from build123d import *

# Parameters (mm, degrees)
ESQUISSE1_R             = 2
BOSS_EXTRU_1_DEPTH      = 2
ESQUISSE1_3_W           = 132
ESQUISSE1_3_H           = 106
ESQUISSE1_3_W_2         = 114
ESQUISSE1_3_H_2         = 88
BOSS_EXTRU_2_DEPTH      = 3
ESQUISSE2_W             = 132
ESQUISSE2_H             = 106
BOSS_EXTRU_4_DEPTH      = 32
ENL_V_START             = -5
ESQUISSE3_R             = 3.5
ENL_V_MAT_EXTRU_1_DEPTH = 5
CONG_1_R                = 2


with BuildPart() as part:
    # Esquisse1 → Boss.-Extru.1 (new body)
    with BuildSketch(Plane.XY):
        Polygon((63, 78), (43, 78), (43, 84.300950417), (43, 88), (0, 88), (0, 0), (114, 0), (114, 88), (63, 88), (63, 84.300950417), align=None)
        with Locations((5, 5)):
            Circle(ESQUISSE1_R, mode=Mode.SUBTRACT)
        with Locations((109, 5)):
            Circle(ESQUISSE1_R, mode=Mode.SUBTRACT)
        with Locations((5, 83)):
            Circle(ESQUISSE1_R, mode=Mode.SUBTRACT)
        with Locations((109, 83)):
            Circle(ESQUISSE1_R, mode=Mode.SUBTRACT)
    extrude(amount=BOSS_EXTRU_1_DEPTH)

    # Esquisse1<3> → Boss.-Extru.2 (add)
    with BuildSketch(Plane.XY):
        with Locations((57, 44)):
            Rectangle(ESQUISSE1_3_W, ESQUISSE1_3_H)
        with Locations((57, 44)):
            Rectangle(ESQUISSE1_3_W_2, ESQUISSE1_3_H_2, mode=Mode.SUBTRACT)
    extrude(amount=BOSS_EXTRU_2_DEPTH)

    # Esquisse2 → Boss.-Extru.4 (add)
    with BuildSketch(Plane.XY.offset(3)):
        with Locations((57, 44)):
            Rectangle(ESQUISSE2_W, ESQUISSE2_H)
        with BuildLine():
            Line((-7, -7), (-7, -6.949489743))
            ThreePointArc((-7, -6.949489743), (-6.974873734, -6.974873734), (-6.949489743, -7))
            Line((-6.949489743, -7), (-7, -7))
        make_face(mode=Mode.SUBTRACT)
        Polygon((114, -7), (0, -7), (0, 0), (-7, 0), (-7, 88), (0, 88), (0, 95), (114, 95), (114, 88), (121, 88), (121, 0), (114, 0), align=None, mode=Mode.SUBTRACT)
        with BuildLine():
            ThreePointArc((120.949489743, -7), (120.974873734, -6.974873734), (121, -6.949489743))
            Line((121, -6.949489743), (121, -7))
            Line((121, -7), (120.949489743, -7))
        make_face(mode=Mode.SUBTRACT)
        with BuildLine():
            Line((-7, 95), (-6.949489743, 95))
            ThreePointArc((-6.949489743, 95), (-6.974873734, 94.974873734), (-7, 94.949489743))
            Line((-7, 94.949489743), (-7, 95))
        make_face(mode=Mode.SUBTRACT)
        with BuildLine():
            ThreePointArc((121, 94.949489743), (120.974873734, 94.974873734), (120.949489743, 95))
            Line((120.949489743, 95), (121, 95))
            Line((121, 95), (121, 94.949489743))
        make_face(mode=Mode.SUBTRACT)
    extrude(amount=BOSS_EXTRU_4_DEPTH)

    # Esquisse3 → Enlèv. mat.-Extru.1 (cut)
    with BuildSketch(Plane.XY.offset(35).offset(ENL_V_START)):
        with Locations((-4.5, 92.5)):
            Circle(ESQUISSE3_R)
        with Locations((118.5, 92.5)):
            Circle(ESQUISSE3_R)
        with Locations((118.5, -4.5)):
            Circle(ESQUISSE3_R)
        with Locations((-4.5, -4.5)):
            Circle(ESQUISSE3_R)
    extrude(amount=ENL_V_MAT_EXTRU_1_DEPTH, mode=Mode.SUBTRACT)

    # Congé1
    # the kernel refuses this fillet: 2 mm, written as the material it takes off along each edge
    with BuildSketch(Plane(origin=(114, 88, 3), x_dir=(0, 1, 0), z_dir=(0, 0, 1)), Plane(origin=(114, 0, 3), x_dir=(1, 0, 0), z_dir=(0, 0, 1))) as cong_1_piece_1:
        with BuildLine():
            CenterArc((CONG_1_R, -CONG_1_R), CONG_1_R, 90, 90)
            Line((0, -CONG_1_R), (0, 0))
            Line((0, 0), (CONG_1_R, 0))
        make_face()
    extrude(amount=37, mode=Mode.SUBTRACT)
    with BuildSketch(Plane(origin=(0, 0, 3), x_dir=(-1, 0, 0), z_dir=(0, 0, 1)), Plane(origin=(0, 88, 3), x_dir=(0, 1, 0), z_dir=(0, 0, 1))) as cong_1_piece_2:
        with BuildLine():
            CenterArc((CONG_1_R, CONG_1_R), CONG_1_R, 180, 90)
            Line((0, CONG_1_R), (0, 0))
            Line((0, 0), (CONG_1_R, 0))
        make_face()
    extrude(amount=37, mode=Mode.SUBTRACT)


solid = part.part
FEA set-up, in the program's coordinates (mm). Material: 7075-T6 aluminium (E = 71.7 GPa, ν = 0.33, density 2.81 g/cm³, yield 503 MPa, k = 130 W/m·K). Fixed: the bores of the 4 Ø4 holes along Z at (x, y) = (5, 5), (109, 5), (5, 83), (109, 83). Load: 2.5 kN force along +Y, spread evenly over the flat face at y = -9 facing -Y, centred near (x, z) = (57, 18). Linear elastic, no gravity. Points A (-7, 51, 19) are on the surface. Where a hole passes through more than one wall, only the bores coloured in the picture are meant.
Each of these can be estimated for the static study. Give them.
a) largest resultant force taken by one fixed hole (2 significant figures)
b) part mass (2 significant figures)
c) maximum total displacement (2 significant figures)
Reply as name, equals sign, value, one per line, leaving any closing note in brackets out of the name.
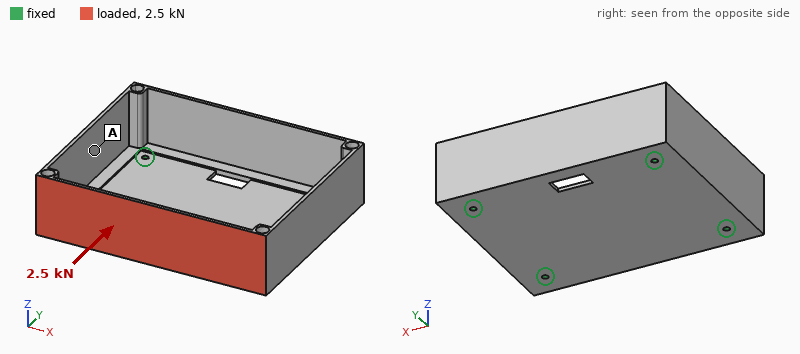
largest resultant force taken by one fixed hole = 720 N
part mass = 190 g
maximum total displacement = 1.8 mm
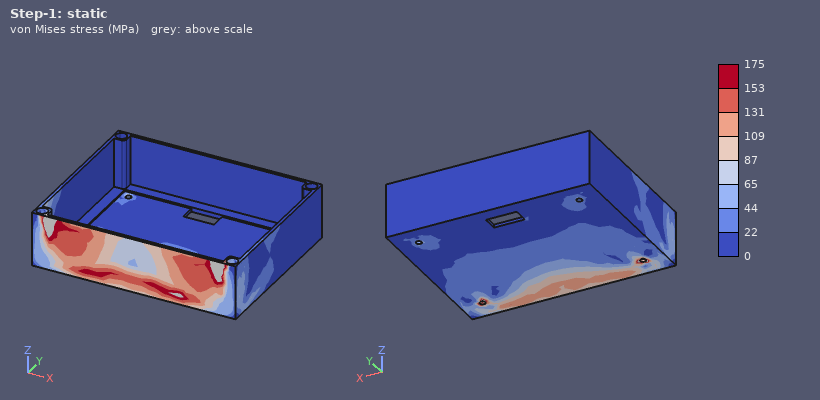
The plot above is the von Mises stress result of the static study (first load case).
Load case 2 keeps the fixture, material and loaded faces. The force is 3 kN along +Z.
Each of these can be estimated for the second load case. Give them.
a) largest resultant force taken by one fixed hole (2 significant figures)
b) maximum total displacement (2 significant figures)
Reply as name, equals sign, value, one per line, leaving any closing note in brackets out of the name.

largest resultant force taken by one fixed hole = 1.8 kN
maximum total displacement = 0.40 mm
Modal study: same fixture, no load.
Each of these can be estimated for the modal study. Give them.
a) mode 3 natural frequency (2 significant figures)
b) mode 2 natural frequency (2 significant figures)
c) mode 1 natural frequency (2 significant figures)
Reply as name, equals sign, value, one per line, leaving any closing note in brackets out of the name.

mode 3 natural frequency = 1800 Hz
mode 2 natural frequency = 1500 Hz
mode 1 natural frequency = 1100 Hz
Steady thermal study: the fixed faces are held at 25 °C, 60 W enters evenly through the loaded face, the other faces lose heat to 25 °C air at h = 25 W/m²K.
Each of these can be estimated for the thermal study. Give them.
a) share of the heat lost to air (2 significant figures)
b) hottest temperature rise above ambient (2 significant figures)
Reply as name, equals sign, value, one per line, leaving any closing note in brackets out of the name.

share of the heat lost to air = 30 %
hottest temperature rise above ambient = 57 K
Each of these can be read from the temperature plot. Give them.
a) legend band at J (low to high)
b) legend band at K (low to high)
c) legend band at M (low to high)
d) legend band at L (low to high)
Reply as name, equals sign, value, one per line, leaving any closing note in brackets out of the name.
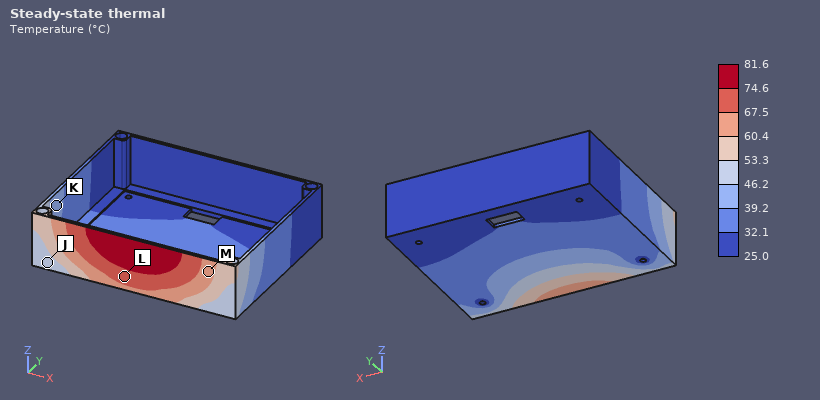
legend band at J = 46.2 to 53.3 °C
legend band at K = 39.2 to 46.2 °C
legend band at M = 60.4 to 67.5 °C
legend band at L = 67.5 to 74.6 °C
